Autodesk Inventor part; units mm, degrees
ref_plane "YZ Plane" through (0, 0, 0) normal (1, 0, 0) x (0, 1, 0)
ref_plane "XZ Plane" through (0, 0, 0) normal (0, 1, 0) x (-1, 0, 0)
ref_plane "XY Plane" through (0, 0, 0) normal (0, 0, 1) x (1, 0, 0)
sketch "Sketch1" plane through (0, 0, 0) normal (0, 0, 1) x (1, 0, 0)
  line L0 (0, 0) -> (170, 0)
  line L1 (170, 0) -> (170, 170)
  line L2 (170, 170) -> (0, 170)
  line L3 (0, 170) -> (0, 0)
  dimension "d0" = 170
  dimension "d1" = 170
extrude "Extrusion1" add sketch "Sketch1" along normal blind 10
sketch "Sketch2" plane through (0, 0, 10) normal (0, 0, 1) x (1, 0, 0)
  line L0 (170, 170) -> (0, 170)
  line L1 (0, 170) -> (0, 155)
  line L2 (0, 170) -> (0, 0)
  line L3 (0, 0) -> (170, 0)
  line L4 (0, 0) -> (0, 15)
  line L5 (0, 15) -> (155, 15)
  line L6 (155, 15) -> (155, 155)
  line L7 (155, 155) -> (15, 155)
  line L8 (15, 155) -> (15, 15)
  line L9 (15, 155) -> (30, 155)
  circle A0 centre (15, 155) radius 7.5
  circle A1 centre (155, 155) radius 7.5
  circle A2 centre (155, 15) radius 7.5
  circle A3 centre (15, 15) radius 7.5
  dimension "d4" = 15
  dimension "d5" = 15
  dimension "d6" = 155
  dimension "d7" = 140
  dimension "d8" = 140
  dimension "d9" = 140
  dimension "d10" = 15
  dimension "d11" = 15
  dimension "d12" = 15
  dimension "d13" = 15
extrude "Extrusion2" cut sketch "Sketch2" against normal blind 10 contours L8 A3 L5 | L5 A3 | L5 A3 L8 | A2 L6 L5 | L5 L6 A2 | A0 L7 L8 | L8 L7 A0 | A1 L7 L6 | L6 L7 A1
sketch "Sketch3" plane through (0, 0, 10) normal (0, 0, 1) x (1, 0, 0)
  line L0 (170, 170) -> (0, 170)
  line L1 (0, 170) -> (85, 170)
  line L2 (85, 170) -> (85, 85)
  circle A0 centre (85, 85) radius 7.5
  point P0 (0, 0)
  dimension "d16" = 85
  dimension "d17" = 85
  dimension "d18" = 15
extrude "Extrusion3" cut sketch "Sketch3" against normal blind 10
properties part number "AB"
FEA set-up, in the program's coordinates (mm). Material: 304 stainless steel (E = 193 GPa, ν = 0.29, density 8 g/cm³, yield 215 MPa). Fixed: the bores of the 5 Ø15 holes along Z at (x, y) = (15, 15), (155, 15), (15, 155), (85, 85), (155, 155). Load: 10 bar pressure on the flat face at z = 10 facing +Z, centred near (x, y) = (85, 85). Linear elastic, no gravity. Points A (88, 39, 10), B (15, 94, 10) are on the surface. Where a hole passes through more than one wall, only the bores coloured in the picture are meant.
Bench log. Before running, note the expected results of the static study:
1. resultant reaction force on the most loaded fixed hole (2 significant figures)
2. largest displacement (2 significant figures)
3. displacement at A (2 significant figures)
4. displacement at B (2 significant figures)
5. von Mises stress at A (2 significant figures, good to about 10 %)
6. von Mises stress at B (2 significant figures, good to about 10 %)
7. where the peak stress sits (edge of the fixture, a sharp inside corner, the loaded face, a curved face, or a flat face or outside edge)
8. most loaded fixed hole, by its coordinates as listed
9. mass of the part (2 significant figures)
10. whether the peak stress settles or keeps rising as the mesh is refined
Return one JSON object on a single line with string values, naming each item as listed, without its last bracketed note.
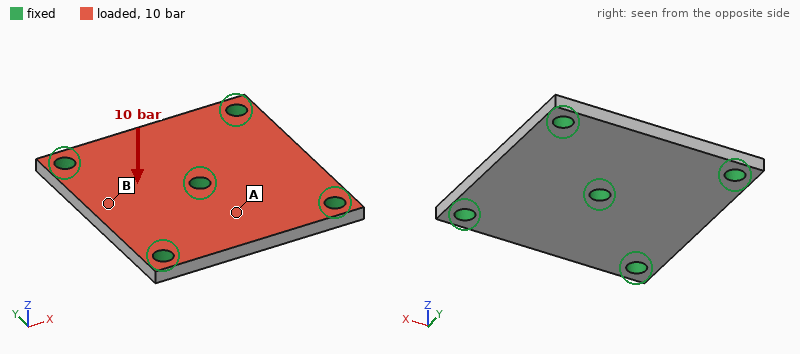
{"resultant reaction force on the most loaded fixed hole": "9.8 kN", "largest displacement": "39 µm", "displacement at A": "24 µm", "displacement at B": "33 µm", "von Mises stress at A": "11 MPa", "von Mises stress at B": "23 MPa", "where the peak stress sits": "edge of the fixture", "most loaded fixed hole, by its coordinates as listed": "(85, 85)", "mass of the part": "2.2 kg", "whether the peak stress settles or keeps rising as the mesh is refined": "keeps rising"}
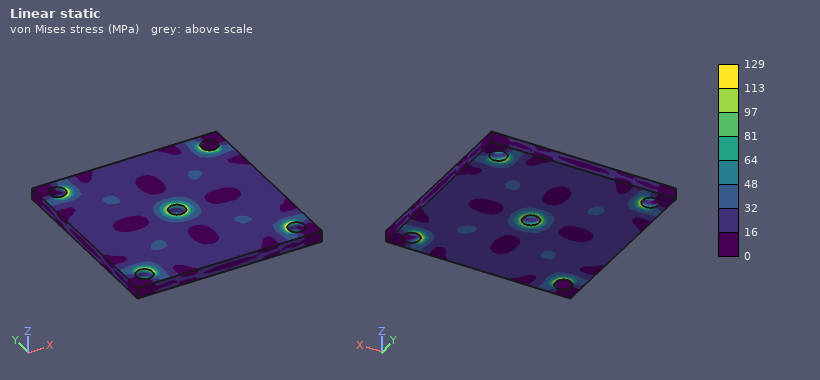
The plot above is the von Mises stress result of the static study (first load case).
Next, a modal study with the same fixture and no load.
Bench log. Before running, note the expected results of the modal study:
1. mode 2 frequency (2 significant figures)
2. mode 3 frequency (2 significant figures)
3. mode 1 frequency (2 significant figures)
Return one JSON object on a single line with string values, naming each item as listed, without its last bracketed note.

{"mode 2 frequency": "3400 Hz", "mode 3 frequency": "3400 Hz", "mode 1 frequency": "3300 Hz"}
